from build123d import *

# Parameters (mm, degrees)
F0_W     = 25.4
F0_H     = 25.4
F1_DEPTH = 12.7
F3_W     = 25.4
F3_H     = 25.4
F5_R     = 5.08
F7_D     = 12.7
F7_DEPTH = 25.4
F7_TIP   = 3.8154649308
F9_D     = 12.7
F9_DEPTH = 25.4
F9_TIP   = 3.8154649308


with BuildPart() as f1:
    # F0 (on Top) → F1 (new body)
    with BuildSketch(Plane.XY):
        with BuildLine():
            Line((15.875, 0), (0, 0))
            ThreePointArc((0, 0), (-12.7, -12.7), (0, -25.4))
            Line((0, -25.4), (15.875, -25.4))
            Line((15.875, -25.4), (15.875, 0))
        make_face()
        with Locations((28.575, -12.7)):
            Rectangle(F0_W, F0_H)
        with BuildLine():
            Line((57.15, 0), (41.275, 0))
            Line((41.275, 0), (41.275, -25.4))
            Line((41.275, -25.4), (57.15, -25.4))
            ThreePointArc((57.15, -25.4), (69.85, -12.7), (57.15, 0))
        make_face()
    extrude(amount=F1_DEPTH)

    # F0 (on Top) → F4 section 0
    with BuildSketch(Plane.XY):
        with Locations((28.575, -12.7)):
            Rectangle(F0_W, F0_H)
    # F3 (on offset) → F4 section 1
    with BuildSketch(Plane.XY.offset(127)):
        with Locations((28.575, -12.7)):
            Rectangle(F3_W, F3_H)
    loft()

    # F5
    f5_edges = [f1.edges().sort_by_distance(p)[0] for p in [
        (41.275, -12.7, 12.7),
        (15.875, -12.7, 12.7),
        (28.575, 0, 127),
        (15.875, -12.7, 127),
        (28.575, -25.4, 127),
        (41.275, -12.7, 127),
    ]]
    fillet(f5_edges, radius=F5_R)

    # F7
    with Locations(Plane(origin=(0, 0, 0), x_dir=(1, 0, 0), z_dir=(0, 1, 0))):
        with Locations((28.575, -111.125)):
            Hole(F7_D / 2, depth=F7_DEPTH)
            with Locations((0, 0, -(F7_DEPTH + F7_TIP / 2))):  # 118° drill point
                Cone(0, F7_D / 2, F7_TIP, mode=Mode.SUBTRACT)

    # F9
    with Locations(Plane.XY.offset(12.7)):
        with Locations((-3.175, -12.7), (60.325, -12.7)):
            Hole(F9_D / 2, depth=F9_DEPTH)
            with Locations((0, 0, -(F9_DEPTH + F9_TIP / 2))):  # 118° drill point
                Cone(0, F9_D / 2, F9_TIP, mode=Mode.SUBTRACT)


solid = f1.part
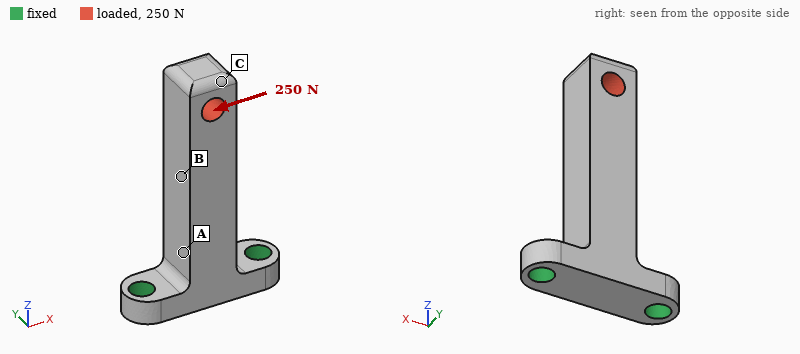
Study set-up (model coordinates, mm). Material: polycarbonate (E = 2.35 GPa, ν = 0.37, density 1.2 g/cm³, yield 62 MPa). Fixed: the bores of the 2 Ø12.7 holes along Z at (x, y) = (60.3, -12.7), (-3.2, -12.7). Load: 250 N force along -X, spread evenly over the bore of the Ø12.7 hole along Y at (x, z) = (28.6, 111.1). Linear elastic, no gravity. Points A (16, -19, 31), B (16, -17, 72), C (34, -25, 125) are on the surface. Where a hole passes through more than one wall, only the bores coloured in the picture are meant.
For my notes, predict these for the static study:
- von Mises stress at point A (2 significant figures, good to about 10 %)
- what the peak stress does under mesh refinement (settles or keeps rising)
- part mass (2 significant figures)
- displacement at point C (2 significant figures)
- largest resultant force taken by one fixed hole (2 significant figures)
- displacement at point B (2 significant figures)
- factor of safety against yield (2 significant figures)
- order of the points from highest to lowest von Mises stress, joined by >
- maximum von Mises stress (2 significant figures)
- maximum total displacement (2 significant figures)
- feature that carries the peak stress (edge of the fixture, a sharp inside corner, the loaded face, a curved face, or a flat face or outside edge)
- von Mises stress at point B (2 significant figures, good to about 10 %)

7.3 MPa
settles
110 g
1.7 mm
610 N
0.72 mm
4.0
A > B > C
15 MPa
1.7 mm
a curved face
3.6 MPa
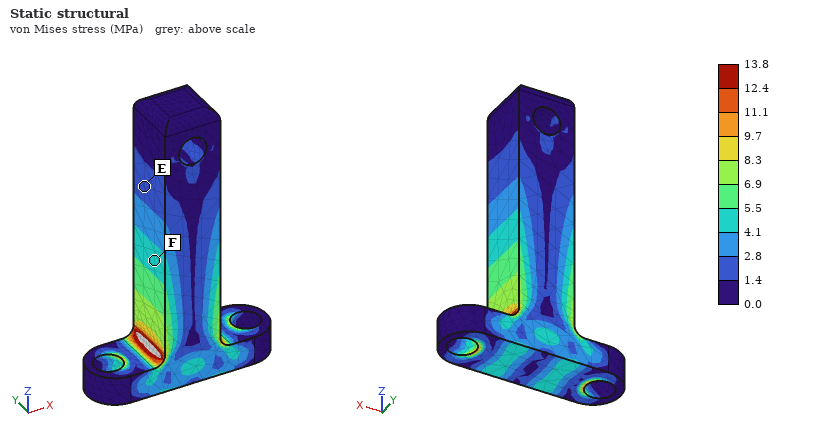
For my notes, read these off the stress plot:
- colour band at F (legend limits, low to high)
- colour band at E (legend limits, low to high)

4.1 to 5.5 MPa
1.4 to 2.8 MPa
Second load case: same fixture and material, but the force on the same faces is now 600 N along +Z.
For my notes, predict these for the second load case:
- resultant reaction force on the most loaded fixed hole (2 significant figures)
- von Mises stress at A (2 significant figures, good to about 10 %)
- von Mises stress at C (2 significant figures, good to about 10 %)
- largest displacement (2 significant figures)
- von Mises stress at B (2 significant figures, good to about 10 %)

320 N
0.87 MPa
0.63 MPa
84 µm
0.93 MPa
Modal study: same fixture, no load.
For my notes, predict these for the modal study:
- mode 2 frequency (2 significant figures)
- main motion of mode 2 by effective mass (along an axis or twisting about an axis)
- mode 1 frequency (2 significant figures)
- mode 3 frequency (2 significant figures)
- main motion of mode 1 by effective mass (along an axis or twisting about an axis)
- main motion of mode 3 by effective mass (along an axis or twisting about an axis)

380 Hz
along X
250 Hz
1700 Hz
along Y
along Y
